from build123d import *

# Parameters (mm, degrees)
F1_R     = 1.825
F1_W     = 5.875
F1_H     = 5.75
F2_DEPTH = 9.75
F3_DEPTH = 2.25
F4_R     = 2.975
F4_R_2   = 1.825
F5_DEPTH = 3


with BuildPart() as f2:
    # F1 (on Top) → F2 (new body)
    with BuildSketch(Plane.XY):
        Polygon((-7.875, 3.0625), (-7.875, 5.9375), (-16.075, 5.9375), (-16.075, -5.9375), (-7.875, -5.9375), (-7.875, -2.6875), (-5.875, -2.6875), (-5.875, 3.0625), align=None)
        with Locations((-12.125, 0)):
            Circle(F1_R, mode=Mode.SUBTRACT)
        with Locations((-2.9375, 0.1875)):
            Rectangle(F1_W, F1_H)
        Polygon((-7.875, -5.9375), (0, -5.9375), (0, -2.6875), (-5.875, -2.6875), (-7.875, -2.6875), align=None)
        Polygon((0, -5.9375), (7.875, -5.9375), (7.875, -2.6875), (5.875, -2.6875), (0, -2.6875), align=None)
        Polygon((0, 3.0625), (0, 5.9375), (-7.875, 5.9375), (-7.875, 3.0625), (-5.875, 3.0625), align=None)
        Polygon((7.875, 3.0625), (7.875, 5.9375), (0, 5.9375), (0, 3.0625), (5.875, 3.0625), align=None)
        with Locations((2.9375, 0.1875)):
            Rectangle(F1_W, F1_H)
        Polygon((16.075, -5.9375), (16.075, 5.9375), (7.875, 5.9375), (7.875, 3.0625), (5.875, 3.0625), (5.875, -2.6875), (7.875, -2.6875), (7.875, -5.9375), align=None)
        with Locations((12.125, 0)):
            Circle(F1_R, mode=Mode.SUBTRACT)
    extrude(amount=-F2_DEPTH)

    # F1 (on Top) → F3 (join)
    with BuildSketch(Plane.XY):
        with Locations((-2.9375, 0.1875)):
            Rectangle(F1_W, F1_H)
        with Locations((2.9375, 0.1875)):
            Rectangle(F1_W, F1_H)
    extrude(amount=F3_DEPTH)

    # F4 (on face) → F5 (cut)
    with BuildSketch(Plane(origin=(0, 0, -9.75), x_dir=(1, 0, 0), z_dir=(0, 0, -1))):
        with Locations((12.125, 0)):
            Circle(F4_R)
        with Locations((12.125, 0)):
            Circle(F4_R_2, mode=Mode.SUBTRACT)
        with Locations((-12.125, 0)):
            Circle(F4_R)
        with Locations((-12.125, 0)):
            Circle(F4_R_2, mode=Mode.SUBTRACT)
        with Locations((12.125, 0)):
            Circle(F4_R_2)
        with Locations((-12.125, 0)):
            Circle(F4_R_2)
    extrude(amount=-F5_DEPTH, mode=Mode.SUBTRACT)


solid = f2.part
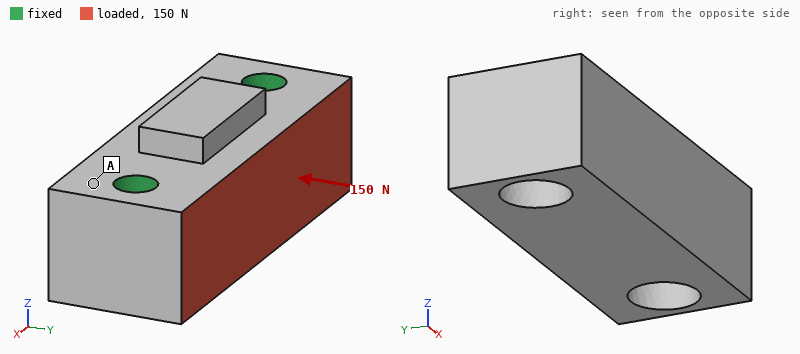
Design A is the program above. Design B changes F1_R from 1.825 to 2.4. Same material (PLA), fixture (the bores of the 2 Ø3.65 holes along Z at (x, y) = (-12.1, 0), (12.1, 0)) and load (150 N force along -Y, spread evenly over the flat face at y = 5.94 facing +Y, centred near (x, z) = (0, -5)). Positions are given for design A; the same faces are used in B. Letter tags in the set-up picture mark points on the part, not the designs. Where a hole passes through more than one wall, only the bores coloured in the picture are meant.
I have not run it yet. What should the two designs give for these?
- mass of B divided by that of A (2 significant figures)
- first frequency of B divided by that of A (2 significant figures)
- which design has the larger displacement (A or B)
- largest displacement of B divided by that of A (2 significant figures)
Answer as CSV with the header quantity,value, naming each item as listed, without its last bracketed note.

quantity,value
mass of B divided by that of A,0.97
first frequency of B divided by that of A,1.1
which design has the larger displacement,A
largest displacement of B divided by that of A,0.80
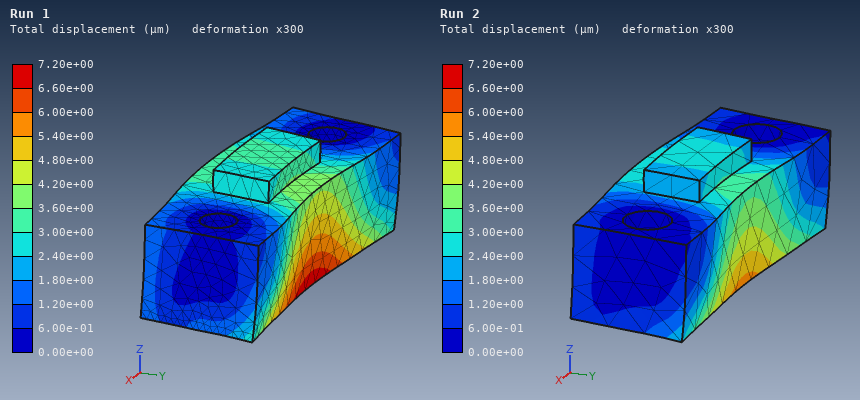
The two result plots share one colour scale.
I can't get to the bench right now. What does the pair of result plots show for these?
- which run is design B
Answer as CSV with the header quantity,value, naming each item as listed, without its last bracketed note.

quantity,value
which run is design B,Run 2
